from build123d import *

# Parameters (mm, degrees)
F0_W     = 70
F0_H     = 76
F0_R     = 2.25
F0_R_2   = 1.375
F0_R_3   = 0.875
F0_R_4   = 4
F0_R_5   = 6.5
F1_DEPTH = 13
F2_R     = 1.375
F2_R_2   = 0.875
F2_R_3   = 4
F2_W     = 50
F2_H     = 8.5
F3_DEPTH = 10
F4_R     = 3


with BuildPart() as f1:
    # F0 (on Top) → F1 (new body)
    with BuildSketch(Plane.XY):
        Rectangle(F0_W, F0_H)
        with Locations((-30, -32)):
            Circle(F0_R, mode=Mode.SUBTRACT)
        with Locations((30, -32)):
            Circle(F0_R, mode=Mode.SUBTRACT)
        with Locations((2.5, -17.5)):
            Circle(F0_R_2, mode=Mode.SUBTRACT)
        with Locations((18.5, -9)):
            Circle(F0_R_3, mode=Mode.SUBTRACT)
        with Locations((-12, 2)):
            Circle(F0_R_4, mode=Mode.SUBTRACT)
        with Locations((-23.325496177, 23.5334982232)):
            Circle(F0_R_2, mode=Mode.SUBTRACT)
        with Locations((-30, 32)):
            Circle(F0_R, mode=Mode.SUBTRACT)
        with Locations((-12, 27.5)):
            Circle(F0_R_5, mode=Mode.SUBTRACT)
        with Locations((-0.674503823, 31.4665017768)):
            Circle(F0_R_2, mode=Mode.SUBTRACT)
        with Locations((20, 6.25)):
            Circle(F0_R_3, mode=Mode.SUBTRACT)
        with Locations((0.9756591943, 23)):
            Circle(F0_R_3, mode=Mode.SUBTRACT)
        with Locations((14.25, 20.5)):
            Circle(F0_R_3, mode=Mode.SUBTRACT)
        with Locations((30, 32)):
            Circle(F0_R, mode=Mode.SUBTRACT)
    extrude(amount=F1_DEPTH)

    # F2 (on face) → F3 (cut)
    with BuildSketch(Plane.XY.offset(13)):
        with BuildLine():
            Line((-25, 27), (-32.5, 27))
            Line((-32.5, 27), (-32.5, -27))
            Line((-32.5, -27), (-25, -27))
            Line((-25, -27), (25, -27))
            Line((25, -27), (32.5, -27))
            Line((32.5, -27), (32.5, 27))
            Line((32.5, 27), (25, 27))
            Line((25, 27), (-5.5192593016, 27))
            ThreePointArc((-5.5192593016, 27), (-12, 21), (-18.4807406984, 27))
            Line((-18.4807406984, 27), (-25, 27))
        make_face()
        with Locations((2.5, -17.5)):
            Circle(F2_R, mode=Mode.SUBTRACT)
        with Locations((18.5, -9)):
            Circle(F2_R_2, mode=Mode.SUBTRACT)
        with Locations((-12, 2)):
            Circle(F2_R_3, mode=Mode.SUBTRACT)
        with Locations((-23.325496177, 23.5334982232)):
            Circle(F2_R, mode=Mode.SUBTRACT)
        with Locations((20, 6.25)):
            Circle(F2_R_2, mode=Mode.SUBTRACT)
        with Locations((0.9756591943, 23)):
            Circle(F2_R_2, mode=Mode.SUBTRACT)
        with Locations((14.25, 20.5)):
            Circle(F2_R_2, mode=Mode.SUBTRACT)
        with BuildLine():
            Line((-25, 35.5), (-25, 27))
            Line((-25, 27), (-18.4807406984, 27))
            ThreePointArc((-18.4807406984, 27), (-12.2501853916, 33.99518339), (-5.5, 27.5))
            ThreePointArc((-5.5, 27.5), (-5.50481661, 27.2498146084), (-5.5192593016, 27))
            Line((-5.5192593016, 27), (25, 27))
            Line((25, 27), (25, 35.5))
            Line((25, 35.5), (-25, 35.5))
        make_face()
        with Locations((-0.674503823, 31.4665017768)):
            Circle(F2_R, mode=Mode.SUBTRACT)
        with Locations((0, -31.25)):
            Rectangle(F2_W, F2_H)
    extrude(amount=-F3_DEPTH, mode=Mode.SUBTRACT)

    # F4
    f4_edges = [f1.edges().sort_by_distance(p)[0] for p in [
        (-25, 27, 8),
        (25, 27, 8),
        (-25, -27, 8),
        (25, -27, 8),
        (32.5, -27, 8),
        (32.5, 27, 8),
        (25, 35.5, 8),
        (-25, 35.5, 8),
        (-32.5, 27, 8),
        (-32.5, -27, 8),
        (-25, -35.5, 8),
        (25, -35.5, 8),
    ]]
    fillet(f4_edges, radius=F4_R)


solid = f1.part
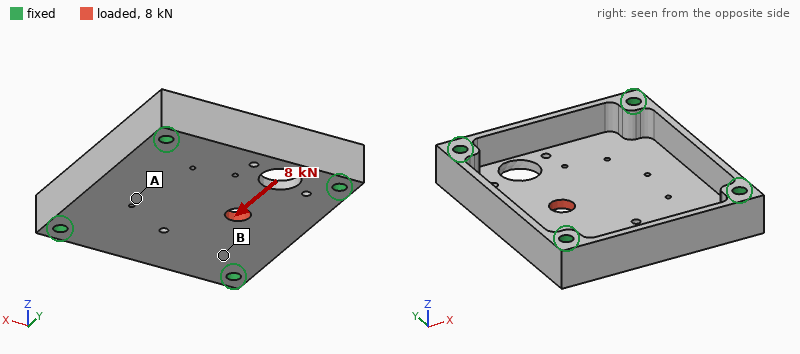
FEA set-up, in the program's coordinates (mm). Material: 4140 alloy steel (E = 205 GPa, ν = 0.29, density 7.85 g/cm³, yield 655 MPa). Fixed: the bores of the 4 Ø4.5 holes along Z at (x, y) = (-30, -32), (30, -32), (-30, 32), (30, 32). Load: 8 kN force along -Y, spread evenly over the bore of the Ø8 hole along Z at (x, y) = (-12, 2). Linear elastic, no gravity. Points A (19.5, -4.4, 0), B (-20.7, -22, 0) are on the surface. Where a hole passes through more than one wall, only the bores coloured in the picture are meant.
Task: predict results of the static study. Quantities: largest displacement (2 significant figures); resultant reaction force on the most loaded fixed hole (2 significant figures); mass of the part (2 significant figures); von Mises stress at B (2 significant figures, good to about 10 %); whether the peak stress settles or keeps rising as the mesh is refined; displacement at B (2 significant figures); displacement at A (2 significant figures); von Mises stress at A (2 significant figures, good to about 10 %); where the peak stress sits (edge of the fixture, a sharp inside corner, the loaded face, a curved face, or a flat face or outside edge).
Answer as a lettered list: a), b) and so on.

a) 12 µm
b) 2.8 kN
c) 190 g
d) 46 MPa
e) keeps rising
f) 3.9 µm
g) 2.6 µm
h) 17 MPa
i) a sharp inside corner
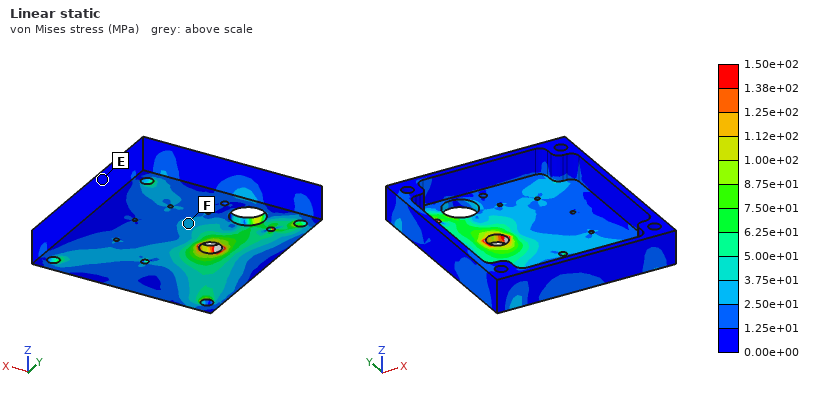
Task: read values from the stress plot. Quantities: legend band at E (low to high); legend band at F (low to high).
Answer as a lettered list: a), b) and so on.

a) 0.00e+00 to 1.25e+01 MPa
b) 2.50e+01 to 3.75e+01 MPa
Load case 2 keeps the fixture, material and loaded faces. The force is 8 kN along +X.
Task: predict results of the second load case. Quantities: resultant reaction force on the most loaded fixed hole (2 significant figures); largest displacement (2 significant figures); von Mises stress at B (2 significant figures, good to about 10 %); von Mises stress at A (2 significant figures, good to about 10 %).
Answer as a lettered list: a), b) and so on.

a) 2.4 kN
b) 15 µm
c) 38 MPa
d) 18 MPa
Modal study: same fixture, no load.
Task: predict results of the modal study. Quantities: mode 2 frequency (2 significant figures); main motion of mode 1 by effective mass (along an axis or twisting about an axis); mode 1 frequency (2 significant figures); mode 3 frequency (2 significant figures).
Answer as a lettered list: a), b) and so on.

a) 7800 Hz
b) along Z
c) 3800 Hz
d) 8000 Hz
